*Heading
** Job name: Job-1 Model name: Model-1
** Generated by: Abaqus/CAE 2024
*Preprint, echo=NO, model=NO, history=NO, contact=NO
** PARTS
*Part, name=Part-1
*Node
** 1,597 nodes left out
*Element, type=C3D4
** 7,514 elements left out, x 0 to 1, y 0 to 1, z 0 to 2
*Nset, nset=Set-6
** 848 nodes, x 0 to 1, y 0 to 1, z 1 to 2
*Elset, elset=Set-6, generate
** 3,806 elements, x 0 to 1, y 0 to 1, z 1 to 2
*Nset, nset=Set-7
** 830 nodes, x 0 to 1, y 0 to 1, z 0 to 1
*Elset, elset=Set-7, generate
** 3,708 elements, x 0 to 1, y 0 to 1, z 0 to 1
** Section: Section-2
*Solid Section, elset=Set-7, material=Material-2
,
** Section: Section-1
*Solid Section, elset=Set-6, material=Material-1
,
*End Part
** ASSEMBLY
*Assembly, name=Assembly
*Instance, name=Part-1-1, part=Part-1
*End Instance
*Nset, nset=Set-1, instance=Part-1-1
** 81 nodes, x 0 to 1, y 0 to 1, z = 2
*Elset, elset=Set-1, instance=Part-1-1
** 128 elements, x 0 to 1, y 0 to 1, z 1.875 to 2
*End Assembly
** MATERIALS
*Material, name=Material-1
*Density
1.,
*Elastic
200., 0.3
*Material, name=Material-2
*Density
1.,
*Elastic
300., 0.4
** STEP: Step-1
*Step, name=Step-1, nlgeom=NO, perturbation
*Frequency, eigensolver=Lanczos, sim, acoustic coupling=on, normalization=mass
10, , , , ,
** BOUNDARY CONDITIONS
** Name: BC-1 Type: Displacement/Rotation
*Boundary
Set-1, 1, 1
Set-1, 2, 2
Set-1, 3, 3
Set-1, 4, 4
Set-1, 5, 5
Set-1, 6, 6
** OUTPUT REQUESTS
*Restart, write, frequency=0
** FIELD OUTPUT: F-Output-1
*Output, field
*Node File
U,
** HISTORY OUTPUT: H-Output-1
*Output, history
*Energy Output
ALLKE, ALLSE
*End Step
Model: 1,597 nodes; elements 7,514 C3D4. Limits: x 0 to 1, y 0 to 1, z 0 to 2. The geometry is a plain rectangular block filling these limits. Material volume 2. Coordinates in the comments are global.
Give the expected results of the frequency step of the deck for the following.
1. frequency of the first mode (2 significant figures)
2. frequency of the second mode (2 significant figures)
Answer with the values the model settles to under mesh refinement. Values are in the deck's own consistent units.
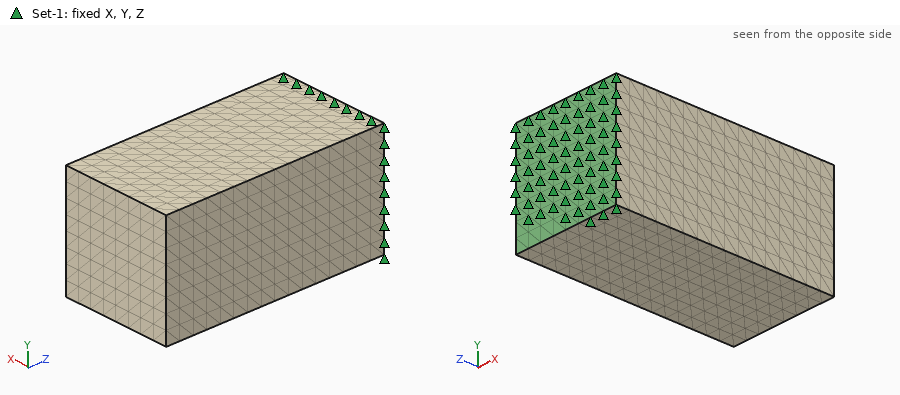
0.50 cycles per unit time
0.50 cycles per unit time
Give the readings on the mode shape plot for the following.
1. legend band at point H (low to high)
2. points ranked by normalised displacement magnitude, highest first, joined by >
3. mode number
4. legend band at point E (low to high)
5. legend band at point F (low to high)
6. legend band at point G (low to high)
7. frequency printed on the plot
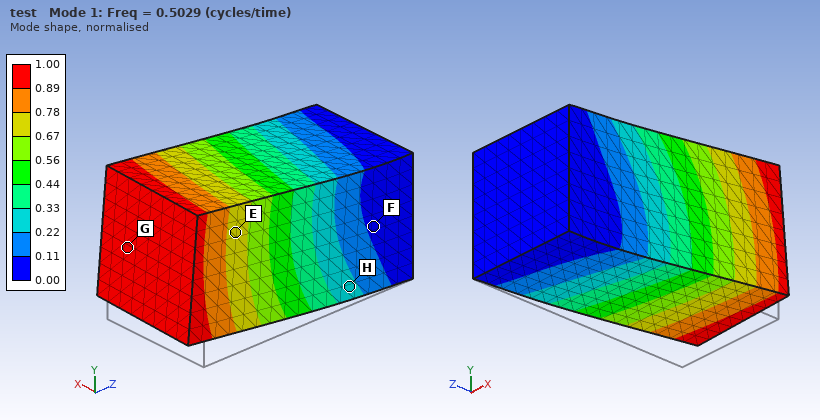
0.22 to 0.33
G > E > H > F
1
0.67 to 0.78
0.00 to 0.11
0.89 to 1.00
0.5029
